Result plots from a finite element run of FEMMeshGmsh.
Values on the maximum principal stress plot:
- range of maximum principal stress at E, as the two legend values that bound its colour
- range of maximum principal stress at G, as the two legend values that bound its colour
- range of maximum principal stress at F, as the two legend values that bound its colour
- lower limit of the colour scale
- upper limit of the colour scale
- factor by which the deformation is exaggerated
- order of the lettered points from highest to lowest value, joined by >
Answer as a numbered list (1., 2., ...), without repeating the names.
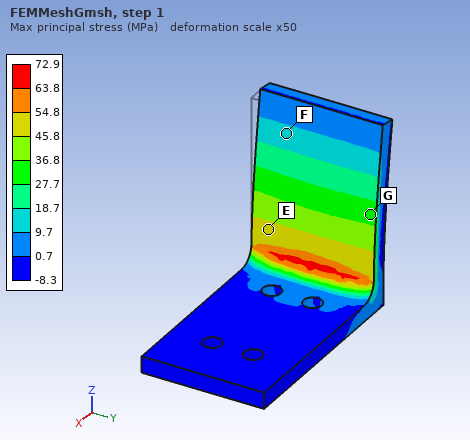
1. 45.8 to 54.8 MPa
2. 27.7 to 36.8 MPa
3. 9.7 to 18.7 MPa
4. -8.3 MPa
5. 72.9 MPa
6. 50
7. E > G > F
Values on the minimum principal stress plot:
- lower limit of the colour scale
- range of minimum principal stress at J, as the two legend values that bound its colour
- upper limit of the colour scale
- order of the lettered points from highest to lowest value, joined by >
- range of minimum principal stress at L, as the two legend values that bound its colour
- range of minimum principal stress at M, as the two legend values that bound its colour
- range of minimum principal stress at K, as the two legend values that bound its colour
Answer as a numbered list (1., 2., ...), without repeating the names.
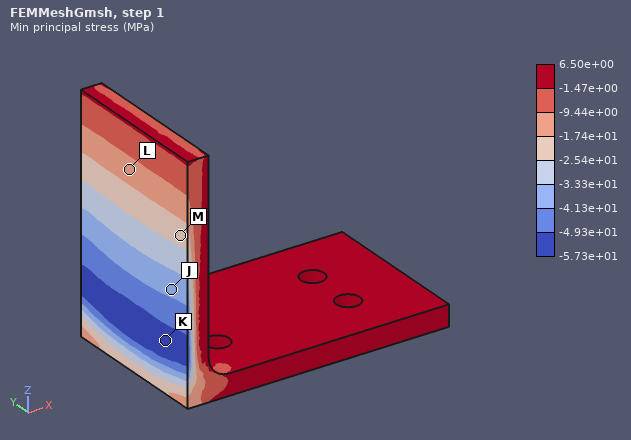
1. -5.73e+01 MPa
2. -4.13e+01 to -3.33e+01 MPa
3. 6.50e+00 MPa
4. L > M > J > K
5. -1.74e+01 to -9.44e+00 MPa
6. -2.54e+01 to -1.74e+01 MPa
7. -5.73e+01 to -4.93e+01 MPa
